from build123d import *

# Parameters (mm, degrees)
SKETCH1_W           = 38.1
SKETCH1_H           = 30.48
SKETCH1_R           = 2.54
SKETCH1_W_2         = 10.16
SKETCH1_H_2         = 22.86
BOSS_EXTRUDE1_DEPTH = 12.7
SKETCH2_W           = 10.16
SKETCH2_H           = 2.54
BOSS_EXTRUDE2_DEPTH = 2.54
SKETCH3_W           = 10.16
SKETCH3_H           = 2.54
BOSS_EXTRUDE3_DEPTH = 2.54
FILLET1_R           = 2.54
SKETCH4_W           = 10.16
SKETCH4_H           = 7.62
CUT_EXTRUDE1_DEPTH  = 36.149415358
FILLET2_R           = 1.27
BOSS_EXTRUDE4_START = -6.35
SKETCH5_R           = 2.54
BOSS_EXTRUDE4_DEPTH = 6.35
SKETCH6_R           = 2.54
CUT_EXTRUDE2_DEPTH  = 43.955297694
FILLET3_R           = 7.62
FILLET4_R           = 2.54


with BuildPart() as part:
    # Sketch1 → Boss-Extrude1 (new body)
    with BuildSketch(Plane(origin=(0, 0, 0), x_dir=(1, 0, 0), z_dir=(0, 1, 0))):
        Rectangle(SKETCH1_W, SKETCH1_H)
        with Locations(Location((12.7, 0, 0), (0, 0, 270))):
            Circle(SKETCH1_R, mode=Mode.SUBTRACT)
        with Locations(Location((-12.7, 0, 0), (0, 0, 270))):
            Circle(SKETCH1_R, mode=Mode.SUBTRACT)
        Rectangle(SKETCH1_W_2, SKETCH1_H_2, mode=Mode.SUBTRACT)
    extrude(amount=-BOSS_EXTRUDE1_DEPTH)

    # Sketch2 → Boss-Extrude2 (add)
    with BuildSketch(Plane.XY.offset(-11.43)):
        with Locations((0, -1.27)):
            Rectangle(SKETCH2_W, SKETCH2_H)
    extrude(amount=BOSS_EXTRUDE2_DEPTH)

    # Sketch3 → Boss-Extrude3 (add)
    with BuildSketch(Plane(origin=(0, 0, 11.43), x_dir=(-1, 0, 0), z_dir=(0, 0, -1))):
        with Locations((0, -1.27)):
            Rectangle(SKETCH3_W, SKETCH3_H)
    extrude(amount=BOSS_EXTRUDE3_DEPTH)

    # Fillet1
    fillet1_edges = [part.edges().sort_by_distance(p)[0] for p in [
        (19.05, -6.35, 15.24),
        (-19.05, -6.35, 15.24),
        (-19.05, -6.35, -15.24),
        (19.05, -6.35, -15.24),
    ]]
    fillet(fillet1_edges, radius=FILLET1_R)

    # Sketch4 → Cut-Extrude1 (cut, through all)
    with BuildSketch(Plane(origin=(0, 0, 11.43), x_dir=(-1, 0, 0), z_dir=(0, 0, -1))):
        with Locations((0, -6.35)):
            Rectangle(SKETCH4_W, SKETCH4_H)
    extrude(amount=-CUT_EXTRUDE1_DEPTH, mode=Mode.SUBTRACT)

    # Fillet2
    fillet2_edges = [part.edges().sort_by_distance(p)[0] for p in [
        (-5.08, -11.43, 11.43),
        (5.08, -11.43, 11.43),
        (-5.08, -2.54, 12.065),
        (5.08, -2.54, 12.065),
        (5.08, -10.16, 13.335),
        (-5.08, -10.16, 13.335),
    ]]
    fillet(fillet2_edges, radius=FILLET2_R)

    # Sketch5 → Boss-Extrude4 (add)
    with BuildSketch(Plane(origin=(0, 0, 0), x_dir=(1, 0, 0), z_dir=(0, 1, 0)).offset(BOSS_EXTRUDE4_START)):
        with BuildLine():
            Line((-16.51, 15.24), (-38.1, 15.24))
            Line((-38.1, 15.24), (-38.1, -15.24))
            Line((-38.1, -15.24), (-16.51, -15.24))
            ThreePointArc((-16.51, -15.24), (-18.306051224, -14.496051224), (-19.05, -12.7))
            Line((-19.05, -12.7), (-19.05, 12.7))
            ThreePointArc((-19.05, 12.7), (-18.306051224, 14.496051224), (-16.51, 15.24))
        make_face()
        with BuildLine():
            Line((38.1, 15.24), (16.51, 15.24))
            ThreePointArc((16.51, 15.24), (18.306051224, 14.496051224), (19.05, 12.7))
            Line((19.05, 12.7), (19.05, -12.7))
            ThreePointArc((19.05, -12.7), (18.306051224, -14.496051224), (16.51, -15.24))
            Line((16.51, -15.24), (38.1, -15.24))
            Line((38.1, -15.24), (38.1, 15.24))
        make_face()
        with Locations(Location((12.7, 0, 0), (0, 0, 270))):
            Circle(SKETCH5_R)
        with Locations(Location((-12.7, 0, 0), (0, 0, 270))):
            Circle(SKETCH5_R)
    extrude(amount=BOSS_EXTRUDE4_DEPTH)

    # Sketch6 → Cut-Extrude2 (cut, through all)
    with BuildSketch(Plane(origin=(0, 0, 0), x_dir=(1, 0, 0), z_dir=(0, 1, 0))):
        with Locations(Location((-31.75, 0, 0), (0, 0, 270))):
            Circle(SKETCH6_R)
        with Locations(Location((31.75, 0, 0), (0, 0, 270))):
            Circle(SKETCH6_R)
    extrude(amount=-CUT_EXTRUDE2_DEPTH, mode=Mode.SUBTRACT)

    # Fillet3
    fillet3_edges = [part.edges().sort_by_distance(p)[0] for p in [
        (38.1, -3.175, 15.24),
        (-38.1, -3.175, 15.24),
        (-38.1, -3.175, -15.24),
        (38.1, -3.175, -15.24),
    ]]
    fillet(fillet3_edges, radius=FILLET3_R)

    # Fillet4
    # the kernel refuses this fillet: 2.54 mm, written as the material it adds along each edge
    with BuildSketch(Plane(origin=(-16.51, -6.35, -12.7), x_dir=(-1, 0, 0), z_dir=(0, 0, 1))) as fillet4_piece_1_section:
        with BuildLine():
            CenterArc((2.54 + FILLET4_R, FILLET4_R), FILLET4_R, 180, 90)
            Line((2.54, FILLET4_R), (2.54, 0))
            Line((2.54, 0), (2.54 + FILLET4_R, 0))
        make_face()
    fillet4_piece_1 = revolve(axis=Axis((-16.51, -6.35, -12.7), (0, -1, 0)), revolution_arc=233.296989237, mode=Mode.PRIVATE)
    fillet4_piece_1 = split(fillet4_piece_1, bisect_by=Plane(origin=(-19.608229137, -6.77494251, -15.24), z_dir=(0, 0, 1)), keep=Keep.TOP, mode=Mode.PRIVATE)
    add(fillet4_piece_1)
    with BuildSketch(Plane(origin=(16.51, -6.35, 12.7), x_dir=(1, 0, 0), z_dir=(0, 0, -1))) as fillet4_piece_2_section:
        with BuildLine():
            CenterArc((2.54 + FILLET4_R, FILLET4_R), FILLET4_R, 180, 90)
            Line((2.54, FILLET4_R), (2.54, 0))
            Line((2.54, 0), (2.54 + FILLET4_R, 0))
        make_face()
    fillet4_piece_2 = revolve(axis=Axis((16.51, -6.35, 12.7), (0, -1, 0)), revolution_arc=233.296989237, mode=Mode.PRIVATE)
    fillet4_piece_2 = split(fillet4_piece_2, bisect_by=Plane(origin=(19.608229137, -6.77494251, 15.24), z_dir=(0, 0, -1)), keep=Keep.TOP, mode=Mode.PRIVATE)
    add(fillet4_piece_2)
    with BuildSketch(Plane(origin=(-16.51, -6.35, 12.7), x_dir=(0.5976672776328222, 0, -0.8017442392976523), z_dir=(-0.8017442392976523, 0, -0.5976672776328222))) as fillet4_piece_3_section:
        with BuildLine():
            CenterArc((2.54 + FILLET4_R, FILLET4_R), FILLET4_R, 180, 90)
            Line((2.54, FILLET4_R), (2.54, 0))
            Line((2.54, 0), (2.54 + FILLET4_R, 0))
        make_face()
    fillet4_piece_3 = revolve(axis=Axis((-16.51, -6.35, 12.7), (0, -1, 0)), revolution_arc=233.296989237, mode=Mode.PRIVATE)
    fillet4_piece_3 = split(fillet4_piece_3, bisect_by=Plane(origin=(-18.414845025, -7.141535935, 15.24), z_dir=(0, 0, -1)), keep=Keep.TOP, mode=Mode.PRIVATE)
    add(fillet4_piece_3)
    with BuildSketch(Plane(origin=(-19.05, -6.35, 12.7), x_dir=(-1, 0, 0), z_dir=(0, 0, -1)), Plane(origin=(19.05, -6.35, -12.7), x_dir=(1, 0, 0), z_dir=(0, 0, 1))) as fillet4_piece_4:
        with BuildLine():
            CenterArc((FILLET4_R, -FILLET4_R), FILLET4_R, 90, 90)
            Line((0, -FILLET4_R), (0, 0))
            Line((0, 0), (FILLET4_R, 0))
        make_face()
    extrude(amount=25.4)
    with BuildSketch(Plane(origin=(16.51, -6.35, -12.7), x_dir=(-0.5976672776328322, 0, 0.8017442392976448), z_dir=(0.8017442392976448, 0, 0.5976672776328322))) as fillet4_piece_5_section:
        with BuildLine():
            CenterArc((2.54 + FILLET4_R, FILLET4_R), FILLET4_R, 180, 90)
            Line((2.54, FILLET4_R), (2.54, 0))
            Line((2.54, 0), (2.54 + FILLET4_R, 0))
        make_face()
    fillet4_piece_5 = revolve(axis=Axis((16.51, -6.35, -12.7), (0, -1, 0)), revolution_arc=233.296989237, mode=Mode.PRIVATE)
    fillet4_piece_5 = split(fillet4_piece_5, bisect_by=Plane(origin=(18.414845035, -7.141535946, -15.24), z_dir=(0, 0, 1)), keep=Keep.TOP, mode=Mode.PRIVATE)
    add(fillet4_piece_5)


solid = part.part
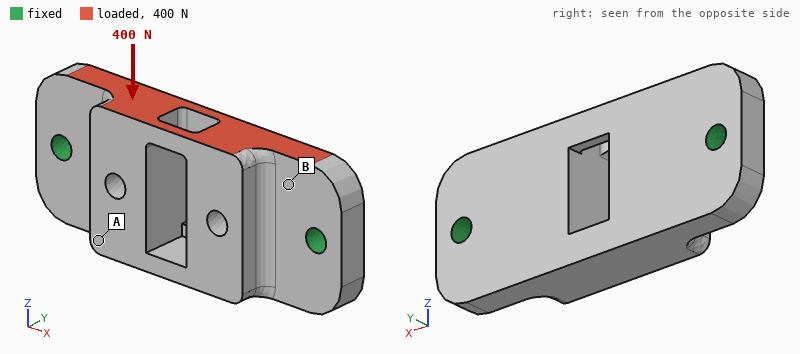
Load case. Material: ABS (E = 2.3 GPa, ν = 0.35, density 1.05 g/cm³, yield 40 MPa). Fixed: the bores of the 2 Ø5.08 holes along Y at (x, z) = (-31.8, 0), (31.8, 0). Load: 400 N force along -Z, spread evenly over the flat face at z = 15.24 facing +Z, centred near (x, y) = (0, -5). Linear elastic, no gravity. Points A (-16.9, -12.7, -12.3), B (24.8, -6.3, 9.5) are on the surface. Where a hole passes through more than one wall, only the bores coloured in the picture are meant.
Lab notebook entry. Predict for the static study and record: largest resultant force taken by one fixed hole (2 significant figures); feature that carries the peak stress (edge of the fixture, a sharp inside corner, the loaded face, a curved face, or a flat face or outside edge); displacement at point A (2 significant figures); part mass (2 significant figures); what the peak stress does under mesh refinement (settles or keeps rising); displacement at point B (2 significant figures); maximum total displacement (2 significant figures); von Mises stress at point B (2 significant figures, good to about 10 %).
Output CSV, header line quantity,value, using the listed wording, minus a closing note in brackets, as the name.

quantity,value
largest resultant force taken by one fixed hole,200 N
feature that carries the peak stress,edge of the fixture
displacement at point A,0.078 mm
part mass,19 g
what the peak stress does under mesh refinement,keeps rising
displacement at point B,0.035 mm
maximum total displacement,0.11 mm
von Mises stress at point B,2.5 MPa
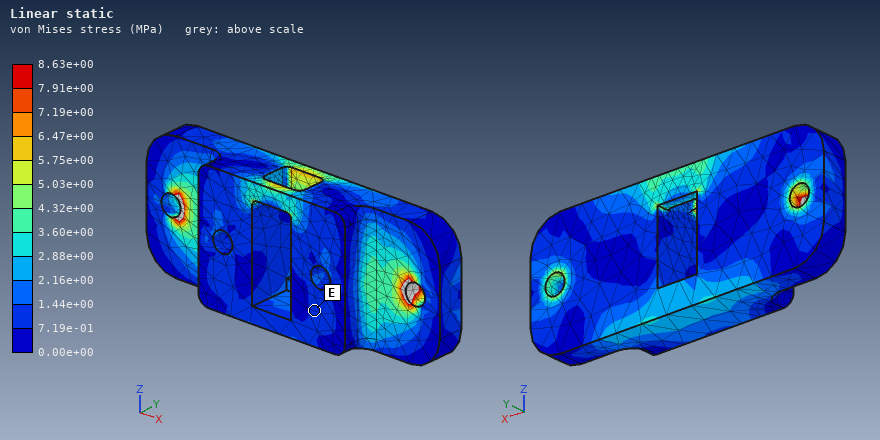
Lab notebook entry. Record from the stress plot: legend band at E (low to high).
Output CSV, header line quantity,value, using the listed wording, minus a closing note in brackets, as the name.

quantity,value
legend band at E,7.19e-01 to 1.44e+00 MPa
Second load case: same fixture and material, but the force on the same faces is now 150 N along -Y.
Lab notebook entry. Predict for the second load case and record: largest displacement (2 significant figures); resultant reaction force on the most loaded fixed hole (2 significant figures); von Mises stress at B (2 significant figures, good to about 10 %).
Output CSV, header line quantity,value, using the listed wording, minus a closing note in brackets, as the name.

quantity,value
largest displacement,0.20 mm
resultant reaction force on the most loaded fixed hole,85 N
von Mises stress at B,2.2 MPa
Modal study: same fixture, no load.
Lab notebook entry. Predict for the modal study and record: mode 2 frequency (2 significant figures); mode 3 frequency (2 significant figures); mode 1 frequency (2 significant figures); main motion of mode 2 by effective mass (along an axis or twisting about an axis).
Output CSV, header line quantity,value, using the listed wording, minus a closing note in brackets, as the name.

quantity,value
mode 2 frequency,2200 Hz
mode 3 frequency,3400 Hz
mode 1 frequency,2200 Hz
main motion of mode 2 by effective mass,along Y
